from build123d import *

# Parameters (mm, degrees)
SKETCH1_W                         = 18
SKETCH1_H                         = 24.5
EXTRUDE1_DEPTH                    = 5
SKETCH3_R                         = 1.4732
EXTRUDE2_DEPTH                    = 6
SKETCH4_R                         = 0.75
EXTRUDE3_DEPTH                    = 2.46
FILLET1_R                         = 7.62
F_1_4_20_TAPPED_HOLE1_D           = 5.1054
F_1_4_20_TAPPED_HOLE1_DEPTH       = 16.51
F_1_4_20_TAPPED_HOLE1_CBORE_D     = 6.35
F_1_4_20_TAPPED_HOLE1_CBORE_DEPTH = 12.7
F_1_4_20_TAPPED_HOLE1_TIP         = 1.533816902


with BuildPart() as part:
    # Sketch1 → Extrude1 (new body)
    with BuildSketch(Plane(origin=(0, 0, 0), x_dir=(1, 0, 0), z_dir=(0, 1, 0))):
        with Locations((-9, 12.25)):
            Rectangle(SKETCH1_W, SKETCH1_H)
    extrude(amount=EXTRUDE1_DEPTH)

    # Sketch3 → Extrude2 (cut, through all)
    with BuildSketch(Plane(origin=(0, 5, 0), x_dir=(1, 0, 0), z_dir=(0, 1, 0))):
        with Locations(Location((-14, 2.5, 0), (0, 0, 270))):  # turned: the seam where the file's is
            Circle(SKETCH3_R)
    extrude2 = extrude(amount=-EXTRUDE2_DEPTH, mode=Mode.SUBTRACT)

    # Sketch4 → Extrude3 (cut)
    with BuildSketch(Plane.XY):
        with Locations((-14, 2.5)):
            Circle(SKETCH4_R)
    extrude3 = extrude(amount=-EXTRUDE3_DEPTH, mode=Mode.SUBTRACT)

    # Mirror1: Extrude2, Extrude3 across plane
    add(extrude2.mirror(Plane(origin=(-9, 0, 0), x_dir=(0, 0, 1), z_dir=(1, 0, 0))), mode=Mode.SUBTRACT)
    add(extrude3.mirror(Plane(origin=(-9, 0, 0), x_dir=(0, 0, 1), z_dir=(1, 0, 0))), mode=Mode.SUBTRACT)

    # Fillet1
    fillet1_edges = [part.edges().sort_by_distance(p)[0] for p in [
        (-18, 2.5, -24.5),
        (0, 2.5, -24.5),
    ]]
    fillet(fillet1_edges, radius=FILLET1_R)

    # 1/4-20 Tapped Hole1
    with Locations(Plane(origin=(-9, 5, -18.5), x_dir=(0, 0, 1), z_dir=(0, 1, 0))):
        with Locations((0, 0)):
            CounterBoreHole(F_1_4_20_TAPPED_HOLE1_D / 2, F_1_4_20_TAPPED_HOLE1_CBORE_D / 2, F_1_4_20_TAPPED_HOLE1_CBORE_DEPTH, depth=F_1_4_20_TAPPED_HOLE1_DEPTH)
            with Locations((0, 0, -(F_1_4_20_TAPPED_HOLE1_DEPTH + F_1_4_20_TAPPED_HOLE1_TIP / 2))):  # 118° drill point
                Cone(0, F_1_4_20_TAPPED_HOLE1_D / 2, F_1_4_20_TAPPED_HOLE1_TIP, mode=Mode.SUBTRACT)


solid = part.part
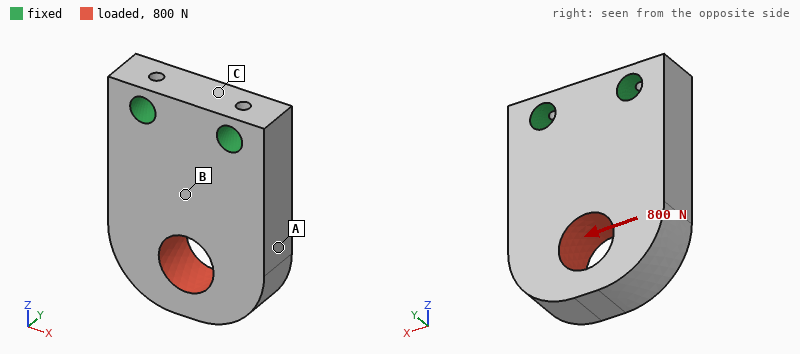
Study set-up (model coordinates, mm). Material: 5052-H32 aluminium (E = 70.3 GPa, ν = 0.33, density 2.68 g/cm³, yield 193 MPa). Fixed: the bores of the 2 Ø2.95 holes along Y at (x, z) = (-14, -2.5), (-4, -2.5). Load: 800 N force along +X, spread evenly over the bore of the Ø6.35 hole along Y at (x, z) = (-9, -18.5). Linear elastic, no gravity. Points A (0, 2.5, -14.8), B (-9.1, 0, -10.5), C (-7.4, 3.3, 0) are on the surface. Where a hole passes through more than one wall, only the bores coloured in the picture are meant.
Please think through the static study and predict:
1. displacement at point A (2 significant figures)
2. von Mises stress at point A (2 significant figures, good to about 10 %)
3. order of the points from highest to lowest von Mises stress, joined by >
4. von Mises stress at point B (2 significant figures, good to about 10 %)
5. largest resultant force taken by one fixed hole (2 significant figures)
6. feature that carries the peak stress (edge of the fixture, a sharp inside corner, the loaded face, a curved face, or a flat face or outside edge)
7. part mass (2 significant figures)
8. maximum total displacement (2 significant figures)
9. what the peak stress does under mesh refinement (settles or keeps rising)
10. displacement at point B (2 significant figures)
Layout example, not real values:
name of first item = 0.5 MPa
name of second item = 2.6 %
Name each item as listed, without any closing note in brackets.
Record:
displacement at point A = 12 µm
von Mises stress at point A = 19 MPa
order of the points from highest to lowest von Mises stress, joined by > = B > A > C
von Mises stress at point B = 31 MPa
largest resultant force taken by one fixed hole = 1.1 kN
feature that carries the peak stress = edge of the fixture
part mass = 5.0 g
maximum total displacement = 21 µm
what the peak stress does under mesh refinement = keeps rising
displacement at point B = 5.5 µm
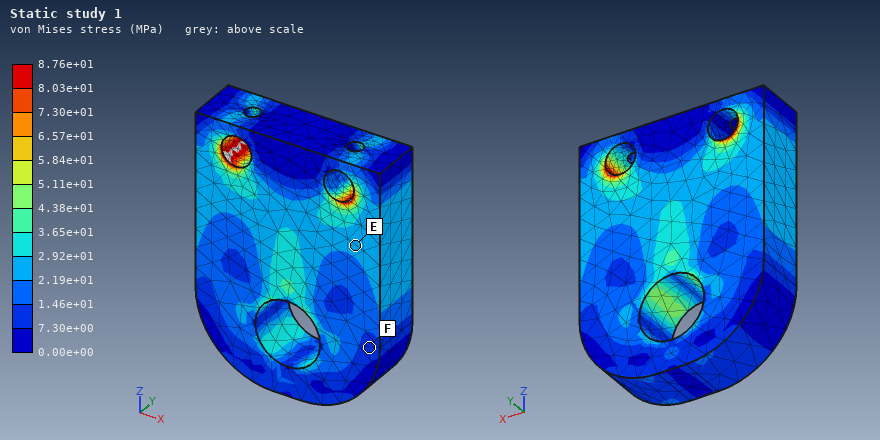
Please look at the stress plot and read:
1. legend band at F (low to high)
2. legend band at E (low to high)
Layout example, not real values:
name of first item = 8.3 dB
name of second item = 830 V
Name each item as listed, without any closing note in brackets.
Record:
legend band at F = 7.30e+00 to 1.46e+01 MPa
legend band at E = 2.19e+01 to 2.92e+01 MPa
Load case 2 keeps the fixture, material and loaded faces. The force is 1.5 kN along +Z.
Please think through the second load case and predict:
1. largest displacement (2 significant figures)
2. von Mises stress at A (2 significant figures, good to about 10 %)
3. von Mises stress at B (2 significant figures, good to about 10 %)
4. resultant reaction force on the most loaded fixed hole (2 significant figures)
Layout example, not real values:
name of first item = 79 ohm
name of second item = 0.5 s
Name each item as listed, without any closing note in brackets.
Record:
largest displacement = 8.3 µm
von Mises stress at A = 7.8 MPa
von Mises stress at B = 17 MPa
resultant reaction force on the most loaded fixed hole = 760 N
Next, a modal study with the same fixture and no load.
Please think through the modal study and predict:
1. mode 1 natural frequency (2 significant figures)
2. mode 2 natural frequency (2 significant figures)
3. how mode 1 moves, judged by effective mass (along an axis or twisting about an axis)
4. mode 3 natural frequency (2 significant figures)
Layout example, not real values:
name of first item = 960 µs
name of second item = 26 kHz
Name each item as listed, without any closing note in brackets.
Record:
mode 1 natural frequency = 10 kHz
mode 2 natural frequency = 23 kHz
how mode 1 moves, judged by effective mass = along Y
mode 3 natural frequency = 24 kHz
